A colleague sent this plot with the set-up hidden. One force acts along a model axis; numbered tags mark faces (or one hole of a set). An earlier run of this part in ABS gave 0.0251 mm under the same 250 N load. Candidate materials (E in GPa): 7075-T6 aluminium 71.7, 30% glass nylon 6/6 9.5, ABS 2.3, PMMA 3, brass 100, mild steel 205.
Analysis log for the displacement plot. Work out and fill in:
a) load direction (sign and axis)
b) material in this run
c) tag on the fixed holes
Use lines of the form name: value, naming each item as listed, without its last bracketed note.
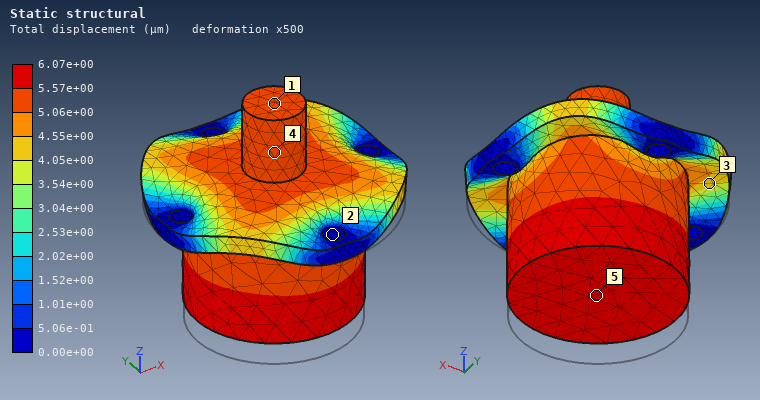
load direction: +Z
material in this run: 30% glass nylon 6/6
tag on the fixed holes: 2
